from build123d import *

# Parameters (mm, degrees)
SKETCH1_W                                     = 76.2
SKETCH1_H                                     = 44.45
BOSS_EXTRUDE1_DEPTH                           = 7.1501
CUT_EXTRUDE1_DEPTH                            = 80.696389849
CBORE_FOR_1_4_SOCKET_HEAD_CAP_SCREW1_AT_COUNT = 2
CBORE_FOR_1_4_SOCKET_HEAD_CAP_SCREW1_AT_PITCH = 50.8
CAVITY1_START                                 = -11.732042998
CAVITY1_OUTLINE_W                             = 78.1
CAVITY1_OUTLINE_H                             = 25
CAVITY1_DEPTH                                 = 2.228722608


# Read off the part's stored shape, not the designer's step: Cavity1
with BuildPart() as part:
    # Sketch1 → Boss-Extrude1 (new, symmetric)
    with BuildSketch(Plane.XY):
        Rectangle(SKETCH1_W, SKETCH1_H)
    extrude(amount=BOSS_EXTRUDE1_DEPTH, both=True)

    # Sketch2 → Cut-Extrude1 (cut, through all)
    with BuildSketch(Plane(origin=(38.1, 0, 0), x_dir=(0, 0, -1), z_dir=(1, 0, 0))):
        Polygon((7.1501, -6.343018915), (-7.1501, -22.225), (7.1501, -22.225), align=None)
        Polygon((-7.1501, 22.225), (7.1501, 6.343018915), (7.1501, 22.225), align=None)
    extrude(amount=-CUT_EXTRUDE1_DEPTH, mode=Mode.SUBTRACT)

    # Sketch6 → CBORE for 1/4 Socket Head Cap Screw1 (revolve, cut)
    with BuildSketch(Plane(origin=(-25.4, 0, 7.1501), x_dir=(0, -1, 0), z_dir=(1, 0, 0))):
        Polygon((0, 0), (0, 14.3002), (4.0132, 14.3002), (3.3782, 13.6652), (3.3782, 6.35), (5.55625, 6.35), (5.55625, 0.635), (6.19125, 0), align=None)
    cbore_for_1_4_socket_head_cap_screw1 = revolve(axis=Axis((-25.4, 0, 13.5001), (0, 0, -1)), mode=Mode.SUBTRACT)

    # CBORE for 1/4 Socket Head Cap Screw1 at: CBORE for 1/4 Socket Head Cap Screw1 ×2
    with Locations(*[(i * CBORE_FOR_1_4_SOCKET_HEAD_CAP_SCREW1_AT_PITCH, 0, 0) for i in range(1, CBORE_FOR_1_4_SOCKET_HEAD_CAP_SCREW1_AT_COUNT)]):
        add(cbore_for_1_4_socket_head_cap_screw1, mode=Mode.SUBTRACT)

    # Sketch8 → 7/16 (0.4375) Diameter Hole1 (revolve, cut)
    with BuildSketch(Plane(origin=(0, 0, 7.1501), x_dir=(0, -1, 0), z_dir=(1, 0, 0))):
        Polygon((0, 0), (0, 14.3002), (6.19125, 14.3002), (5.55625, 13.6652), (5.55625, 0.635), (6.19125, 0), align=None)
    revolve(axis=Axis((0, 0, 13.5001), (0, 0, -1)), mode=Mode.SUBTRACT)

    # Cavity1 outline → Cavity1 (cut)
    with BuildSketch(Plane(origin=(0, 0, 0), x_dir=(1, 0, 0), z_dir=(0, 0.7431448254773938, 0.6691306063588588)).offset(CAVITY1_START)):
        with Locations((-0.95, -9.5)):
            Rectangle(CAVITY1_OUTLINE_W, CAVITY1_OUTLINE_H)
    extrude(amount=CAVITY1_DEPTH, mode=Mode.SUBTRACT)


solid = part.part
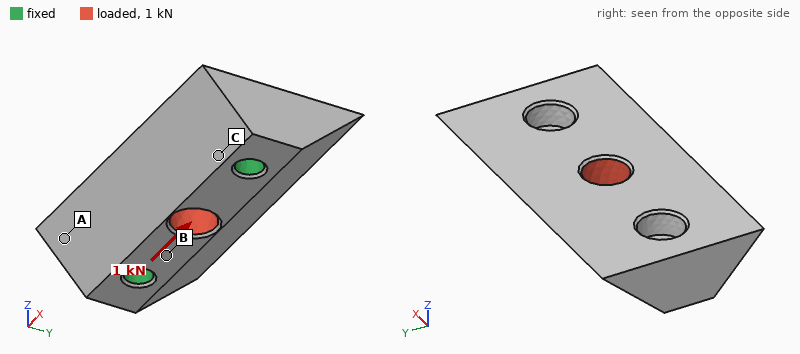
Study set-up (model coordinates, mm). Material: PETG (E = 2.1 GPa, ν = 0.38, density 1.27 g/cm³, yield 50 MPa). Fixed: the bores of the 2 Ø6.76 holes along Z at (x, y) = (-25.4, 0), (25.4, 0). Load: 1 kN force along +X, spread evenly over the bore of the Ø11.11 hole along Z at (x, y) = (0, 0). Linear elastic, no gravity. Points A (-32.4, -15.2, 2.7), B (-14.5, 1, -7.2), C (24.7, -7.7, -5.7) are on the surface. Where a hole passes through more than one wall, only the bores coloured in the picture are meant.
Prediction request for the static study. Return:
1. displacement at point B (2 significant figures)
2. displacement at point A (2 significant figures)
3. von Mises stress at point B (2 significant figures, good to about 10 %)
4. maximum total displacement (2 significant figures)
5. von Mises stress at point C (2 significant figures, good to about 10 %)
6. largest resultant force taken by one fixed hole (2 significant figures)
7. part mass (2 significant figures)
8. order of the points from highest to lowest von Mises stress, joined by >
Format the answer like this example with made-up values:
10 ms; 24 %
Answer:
12 µm; 15 µm; 3.2 MPa; 31 µm; 1.4 MPa; 500 N; 33 g; B > C > A
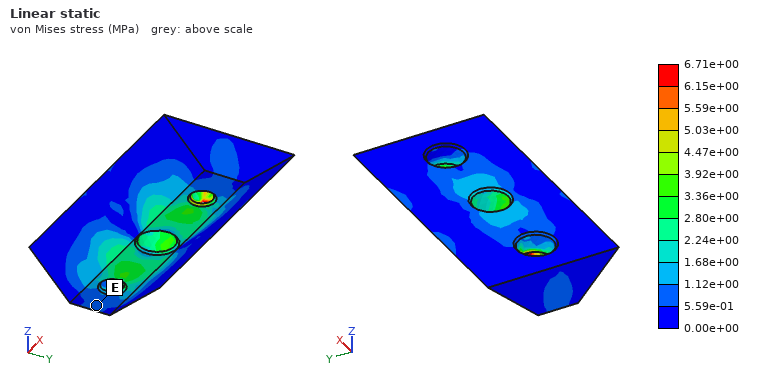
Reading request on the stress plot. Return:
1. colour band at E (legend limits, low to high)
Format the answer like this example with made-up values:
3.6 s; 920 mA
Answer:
5.59e-01 to 1.12e+00 MPa
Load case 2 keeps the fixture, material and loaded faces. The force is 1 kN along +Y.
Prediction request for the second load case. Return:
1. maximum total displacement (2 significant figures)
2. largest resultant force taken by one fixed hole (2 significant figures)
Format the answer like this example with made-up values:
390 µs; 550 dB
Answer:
0.12 mm; 500 N
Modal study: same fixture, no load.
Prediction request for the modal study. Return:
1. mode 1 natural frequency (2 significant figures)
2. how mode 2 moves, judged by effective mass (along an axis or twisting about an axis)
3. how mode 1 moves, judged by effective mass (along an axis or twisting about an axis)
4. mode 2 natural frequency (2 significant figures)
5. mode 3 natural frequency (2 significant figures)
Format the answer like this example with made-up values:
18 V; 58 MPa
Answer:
2800 Hz; along Z; along Y; 3800 Hz; 4300 Hz
